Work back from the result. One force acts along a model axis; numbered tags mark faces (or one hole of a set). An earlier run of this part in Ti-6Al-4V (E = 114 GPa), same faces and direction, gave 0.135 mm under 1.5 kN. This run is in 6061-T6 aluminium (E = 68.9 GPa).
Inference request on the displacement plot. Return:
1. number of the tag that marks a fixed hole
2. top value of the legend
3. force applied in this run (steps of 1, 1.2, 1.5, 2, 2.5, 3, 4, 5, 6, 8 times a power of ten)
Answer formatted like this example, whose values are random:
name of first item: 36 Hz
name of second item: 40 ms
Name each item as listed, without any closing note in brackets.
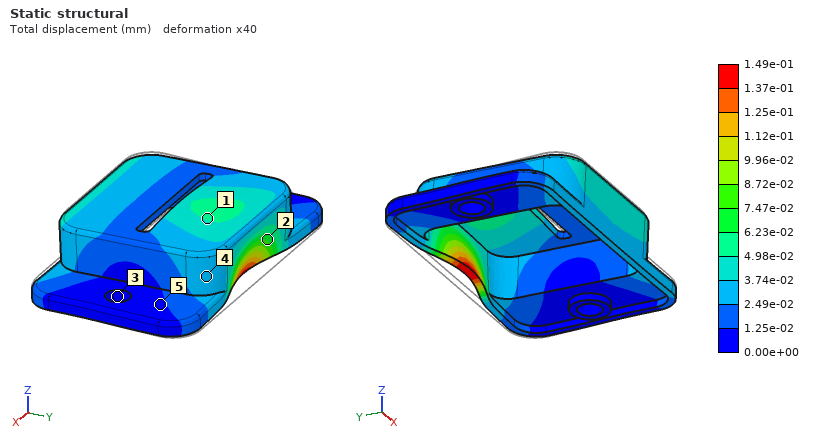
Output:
number of the tag that marks a fixed hole: 3
top value of the legend: 1.49e-01 mm
force applied in this run: 1 kN
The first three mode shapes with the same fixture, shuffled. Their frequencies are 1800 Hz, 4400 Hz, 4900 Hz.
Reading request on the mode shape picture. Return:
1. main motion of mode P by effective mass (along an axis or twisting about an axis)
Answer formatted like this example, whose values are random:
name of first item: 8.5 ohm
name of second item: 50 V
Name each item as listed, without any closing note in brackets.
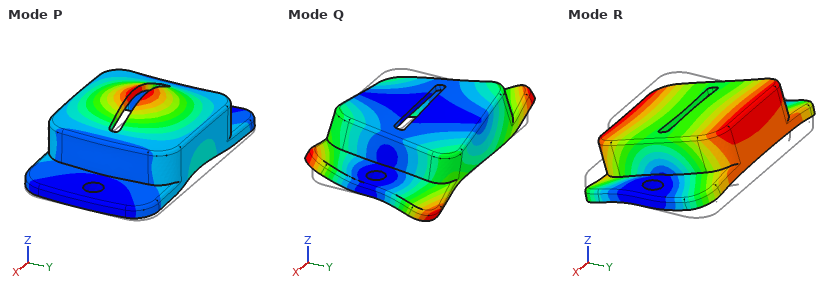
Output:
main motion of mode P by effective mass: along Z
